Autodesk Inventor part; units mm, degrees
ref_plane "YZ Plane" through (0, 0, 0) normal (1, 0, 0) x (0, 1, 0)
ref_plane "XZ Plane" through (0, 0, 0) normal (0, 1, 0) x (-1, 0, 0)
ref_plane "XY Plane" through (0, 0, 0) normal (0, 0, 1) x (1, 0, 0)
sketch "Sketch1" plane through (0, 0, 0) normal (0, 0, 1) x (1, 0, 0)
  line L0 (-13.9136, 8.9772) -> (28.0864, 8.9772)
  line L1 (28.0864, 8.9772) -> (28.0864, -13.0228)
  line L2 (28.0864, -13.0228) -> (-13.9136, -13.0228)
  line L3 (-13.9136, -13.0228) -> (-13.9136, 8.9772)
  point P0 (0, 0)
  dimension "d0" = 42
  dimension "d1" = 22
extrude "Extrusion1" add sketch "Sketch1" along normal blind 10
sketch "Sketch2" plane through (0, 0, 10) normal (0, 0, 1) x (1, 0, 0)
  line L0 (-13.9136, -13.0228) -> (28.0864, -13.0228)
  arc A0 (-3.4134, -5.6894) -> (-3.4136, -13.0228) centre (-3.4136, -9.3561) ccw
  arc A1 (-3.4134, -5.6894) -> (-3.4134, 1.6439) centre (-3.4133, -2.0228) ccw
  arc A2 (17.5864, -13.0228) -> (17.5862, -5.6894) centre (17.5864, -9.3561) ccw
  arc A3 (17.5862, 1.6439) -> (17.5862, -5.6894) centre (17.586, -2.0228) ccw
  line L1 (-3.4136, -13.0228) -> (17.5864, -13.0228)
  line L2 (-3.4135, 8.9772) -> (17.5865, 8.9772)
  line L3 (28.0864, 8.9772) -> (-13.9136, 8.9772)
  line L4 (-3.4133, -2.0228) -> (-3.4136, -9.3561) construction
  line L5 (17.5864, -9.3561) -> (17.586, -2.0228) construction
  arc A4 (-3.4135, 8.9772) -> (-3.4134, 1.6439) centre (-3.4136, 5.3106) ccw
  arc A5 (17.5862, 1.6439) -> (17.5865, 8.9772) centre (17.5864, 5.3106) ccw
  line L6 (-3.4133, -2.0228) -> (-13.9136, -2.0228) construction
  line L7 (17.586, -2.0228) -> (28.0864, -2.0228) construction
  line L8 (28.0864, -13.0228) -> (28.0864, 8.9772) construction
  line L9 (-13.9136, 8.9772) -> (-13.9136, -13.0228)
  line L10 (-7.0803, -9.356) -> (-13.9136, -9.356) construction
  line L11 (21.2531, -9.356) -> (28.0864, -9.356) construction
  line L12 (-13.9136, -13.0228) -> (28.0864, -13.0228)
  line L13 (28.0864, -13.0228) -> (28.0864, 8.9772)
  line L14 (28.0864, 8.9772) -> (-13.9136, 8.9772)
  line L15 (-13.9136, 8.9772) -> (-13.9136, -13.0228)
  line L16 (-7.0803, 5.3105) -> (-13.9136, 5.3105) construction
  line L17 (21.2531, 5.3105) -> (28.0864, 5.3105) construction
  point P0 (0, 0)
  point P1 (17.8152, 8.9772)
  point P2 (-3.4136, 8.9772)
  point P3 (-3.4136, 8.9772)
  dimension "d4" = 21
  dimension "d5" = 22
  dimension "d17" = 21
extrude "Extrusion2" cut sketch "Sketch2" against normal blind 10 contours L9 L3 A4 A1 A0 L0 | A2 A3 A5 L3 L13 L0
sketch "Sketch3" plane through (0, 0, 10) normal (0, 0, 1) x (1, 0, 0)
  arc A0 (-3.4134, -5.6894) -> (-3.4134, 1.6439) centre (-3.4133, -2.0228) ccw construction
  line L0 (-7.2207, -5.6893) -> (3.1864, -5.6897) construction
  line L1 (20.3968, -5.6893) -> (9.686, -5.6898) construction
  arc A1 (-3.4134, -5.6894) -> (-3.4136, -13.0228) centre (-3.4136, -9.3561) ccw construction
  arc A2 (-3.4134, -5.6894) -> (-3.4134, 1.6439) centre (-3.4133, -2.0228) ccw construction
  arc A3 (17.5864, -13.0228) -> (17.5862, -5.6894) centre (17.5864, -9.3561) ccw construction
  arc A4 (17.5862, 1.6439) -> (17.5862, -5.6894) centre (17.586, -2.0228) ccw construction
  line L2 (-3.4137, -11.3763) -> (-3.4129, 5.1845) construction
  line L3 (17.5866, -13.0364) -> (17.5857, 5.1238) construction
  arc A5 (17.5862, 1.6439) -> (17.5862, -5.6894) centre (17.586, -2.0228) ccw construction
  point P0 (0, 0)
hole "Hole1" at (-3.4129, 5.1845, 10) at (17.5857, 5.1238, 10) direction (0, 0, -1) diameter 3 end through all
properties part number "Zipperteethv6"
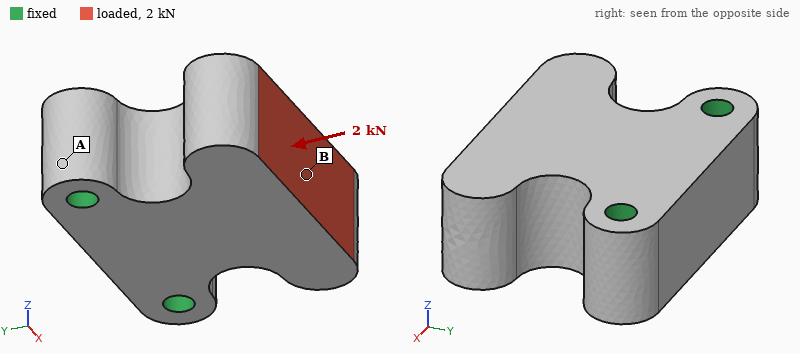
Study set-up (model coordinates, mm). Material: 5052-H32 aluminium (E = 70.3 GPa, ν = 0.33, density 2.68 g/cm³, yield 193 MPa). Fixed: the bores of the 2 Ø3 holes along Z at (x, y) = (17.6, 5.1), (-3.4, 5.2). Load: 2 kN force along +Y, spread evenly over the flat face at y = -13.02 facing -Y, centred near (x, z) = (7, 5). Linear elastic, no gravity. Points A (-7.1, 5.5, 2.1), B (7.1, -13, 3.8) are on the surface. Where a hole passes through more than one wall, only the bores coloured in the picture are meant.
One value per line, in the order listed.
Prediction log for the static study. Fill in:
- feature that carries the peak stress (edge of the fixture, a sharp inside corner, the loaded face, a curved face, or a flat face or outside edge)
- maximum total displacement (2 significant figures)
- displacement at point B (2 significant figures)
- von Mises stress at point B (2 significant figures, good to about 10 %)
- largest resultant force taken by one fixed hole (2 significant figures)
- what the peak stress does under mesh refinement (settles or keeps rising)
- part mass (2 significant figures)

edge of the fixture
6.5 µm
5.3 µm
15 MPa
1.1 kN
keeps rising
13 g
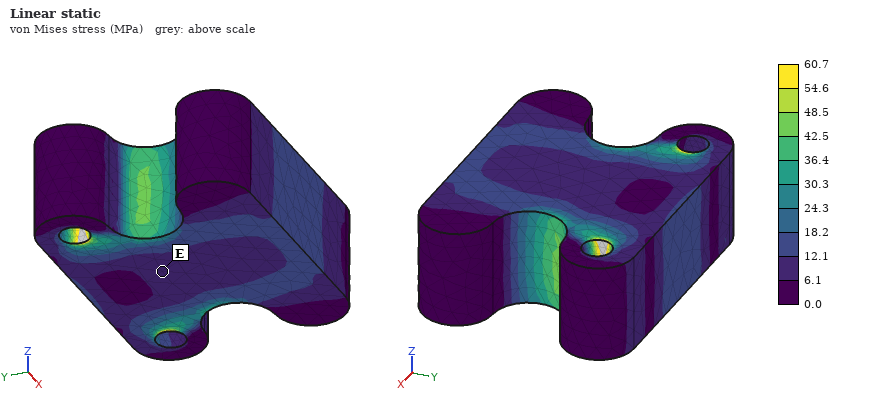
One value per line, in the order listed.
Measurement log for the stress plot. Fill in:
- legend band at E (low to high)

6.1 to 12.1 MPa
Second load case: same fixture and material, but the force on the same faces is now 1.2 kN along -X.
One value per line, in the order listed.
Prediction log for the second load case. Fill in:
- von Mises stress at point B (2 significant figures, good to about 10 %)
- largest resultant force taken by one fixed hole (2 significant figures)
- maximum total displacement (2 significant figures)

10.0 MPa
1.3 kN
22 µm
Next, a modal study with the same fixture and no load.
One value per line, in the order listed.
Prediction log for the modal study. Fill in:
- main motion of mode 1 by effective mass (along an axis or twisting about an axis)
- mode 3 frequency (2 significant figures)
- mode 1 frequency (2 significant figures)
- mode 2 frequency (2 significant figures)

along Z
21 kHz
12 kHz
20 kHz
